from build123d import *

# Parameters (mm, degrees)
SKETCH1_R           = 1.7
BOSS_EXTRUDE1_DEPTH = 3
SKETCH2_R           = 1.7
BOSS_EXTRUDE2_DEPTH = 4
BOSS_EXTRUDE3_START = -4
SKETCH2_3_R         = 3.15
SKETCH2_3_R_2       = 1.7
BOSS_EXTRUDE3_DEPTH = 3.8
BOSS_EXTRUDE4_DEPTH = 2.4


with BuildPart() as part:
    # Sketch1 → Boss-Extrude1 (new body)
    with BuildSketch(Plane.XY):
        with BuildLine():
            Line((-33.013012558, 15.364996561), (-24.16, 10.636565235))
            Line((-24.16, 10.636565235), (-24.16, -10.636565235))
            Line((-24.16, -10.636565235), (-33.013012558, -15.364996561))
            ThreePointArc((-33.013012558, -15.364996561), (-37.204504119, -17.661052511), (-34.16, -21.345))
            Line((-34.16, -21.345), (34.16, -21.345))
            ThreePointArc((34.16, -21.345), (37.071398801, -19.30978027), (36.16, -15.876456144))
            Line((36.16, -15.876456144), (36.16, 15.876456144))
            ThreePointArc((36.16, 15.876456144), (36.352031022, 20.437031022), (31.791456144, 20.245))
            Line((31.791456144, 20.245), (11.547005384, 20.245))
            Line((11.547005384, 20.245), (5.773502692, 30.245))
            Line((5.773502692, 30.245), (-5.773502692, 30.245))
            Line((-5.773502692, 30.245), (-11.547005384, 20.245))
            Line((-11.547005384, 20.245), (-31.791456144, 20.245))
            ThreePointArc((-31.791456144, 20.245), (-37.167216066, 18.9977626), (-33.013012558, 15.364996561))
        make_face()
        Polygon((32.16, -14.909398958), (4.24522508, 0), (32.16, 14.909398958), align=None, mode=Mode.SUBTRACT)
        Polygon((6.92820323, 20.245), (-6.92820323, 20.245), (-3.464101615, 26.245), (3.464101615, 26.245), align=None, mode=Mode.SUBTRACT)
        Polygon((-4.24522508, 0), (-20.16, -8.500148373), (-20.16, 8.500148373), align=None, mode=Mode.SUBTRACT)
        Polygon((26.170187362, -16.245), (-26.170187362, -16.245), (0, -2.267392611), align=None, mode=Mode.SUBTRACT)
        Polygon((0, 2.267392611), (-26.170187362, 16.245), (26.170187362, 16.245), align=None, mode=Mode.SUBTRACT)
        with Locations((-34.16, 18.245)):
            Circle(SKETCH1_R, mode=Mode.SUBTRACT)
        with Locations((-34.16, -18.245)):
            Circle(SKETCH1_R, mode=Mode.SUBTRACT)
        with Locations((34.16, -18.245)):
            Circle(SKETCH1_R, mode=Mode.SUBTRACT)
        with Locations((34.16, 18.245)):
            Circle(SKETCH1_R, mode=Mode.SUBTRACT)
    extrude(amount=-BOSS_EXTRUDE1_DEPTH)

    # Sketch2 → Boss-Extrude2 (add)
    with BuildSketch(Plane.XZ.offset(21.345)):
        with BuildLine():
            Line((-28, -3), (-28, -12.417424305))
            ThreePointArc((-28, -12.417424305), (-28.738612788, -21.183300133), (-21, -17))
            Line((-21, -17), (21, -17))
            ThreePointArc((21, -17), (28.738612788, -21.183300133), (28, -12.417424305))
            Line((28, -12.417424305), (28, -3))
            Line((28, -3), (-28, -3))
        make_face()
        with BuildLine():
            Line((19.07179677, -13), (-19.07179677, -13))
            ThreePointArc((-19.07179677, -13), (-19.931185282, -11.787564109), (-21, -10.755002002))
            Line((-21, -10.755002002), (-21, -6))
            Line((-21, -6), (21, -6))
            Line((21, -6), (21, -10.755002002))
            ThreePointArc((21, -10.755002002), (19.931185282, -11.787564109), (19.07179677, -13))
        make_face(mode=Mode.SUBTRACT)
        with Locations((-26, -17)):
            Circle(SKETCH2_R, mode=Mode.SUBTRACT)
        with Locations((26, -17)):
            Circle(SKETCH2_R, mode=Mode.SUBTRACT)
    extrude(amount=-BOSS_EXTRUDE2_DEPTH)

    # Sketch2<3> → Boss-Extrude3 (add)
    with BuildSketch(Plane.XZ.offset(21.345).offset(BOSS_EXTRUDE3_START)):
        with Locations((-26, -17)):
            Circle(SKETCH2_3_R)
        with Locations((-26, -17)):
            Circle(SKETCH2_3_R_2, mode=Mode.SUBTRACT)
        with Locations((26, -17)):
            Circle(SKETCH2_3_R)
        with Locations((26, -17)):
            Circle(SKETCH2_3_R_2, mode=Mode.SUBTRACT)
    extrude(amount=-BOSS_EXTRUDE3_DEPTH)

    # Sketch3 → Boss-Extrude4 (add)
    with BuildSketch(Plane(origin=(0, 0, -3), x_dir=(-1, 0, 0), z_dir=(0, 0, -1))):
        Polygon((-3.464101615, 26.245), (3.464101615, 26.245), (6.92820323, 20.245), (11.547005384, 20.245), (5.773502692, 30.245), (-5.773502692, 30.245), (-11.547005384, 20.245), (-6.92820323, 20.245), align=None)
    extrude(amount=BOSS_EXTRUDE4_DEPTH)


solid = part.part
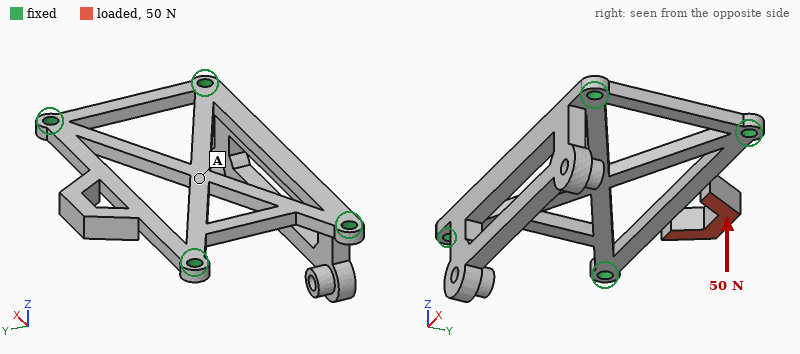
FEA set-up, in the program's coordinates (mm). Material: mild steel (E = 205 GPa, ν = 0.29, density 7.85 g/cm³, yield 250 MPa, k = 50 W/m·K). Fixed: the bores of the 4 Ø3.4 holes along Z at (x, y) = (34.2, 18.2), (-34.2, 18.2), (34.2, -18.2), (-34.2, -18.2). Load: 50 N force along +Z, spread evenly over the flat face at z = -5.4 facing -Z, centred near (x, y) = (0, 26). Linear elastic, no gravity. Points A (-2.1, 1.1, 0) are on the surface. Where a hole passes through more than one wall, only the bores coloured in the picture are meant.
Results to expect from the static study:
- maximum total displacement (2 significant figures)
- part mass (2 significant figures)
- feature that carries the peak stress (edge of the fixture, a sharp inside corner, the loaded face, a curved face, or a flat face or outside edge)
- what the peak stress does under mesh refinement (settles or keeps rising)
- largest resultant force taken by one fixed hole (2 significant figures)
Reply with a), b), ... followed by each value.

a) 49 µm
b) 57 g
c) edge of the fixture
d) keeps rising
e) 26 N
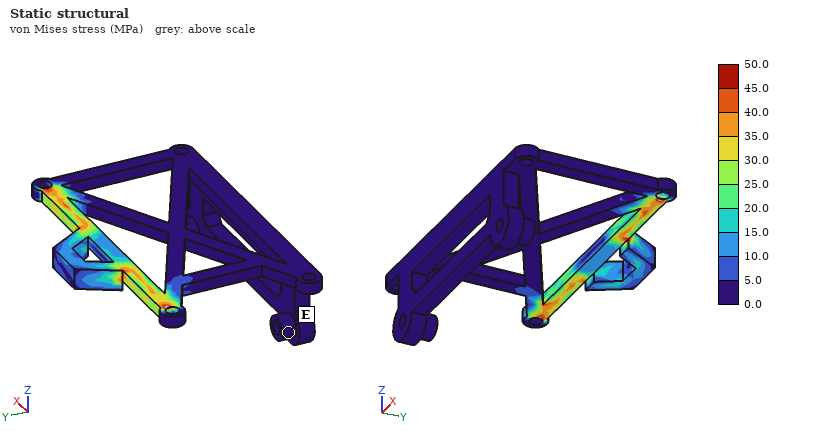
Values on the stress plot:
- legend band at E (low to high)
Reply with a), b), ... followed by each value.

a) 0.0 to 5.0 MPa
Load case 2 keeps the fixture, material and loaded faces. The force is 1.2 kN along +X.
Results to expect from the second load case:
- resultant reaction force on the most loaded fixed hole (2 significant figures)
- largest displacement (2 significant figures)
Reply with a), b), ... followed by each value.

a) 610 N
b) 50 µm
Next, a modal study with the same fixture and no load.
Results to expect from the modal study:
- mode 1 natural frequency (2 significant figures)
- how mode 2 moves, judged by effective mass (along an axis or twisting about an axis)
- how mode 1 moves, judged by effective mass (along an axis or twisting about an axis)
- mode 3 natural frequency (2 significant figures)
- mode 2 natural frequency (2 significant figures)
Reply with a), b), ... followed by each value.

a) 2400 Hz
b) along Y
c) along Z
d) 3500 Hz
e) 2700 Hz
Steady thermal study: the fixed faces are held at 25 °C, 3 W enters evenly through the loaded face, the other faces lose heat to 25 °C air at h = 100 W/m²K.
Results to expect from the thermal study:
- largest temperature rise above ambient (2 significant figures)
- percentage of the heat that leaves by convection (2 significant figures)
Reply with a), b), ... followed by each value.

a) 28 K
b) 73 %
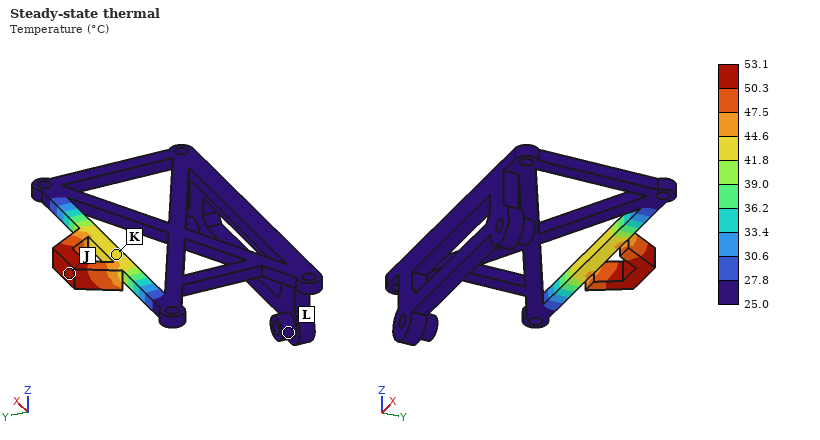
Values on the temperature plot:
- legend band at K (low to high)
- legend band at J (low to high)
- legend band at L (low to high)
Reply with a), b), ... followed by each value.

a) 41.8 to 44.6 °C
b) 50.3 to 53.1 °C
c) 25.0 to 27.8 °C
